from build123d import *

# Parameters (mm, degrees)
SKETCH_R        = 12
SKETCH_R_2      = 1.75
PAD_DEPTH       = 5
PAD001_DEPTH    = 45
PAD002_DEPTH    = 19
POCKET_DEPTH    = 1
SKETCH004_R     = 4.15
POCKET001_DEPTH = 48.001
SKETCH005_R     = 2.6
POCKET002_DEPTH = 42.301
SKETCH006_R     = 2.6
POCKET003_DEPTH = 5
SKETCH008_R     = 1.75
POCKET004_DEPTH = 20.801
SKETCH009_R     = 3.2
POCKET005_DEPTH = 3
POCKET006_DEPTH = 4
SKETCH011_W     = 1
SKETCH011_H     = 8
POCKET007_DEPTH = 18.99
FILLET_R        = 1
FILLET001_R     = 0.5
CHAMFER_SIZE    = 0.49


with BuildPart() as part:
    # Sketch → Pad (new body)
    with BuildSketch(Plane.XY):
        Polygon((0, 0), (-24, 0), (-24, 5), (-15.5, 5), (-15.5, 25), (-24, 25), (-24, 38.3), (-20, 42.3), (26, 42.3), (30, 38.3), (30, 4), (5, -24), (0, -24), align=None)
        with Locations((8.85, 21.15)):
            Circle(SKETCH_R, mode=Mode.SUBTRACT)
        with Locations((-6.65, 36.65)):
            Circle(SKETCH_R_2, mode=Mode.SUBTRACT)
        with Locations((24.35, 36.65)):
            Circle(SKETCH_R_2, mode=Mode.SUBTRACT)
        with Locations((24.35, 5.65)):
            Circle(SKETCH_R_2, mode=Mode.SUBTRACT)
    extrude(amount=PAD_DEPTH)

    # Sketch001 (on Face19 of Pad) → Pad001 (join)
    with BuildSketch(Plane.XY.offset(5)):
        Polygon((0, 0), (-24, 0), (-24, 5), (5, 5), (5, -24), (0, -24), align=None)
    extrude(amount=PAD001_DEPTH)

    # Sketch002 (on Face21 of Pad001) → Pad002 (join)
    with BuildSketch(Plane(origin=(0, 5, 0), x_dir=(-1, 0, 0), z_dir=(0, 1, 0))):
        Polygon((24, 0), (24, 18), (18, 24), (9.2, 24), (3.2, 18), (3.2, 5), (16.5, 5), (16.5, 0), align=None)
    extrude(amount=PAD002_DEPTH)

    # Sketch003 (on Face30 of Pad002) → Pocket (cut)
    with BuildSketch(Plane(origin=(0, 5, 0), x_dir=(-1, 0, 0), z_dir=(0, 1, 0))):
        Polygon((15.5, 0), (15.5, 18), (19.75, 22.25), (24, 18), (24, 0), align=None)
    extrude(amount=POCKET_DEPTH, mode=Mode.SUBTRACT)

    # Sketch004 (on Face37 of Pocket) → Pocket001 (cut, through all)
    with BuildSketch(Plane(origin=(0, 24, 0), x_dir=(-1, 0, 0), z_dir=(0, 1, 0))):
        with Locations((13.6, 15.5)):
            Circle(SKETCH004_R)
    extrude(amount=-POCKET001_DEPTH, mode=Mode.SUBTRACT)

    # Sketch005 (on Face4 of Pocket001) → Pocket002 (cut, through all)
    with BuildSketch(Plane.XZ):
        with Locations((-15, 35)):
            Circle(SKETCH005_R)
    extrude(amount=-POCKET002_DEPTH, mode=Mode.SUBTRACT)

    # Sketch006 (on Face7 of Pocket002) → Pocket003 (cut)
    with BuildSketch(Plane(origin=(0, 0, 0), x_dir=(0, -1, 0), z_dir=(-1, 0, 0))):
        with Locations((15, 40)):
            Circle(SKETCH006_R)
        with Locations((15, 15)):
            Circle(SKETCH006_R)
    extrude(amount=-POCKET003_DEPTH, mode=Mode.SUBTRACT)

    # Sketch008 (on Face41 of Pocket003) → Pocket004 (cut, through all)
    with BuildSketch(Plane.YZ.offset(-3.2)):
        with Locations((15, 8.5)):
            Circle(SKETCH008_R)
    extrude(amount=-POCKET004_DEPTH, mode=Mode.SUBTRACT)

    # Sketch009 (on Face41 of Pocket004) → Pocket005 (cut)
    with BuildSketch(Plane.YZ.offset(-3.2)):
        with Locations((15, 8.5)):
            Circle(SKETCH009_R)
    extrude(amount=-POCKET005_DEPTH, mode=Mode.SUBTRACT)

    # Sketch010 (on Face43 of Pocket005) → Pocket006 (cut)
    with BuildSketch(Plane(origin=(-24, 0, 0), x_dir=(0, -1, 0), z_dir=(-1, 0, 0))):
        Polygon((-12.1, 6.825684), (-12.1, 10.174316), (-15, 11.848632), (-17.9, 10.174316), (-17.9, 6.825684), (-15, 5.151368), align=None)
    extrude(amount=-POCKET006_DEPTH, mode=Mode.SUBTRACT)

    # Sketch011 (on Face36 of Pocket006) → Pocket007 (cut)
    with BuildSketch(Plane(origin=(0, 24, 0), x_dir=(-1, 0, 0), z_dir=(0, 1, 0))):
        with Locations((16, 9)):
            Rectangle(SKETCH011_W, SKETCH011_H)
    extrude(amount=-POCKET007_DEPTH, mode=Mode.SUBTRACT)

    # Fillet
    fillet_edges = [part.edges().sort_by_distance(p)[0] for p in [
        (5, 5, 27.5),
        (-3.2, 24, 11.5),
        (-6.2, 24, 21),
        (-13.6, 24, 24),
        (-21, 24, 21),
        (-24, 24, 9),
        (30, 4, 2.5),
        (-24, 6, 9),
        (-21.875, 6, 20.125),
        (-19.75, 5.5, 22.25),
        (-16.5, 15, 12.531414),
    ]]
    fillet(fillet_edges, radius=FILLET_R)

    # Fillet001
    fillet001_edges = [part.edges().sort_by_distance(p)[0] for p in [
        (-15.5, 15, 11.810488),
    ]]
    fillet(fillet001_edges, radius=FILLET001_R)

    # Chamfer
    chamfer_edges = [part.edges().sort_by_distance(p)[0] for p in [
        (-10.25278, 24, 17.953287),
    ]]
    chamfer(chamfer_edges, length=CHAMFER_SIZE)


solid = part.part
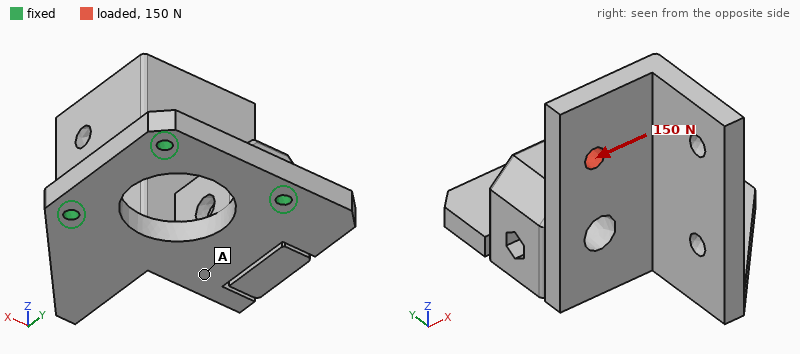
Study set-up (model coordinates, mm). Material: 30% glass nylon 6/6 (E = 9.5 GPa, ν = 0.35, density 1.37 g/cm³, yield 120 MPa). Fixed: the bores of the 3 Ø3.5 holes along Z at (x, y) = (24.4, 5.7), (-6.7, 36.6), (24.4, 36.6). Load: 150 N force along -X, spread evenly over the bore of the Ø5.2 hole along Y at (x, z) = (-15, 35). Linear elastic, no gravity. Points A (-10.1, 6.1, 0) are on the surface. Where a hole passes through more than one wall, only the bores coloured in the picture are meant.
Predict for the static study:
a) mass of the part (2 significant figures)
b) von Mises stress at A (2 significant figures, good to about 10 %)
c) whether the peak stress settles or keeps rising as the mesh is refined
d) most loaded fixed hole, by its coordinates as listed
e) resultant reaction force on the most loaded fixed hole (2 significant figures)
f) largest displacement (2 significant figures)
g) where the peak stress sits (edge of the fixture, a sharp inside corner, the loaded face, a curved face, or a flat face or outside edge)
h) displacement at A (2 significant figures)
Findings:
37 g
4.7 MPa
keeps rising
(24.4, 5.7)
140 N
1.1 mm
edge of the fixture
0.28 mm
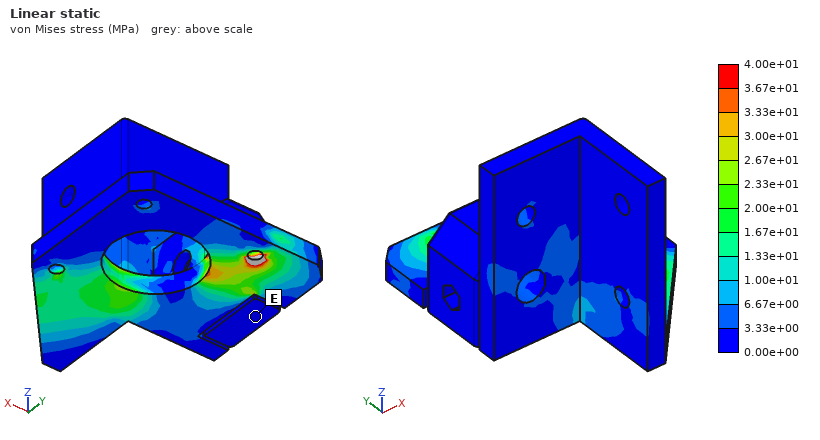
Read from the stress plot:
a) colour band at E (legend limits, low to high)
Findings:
0.00e+00 to 3.33e+00 MPa
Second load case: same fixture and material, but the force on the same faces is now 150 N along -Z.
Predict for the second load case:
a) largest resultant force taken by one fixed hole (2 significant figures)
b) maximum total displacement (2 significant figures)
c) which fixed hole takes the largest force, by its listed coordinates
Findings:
100 N
0.94 mm
(-6.7, 36.6)
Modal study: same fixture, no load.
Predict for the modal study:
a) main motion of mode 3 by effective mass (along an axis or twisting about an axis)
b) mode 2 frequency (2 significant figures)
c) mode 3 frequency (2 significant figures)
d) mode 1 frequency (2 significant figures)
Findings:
along Z
1200 Hz
2000 Hz
480 Hz
